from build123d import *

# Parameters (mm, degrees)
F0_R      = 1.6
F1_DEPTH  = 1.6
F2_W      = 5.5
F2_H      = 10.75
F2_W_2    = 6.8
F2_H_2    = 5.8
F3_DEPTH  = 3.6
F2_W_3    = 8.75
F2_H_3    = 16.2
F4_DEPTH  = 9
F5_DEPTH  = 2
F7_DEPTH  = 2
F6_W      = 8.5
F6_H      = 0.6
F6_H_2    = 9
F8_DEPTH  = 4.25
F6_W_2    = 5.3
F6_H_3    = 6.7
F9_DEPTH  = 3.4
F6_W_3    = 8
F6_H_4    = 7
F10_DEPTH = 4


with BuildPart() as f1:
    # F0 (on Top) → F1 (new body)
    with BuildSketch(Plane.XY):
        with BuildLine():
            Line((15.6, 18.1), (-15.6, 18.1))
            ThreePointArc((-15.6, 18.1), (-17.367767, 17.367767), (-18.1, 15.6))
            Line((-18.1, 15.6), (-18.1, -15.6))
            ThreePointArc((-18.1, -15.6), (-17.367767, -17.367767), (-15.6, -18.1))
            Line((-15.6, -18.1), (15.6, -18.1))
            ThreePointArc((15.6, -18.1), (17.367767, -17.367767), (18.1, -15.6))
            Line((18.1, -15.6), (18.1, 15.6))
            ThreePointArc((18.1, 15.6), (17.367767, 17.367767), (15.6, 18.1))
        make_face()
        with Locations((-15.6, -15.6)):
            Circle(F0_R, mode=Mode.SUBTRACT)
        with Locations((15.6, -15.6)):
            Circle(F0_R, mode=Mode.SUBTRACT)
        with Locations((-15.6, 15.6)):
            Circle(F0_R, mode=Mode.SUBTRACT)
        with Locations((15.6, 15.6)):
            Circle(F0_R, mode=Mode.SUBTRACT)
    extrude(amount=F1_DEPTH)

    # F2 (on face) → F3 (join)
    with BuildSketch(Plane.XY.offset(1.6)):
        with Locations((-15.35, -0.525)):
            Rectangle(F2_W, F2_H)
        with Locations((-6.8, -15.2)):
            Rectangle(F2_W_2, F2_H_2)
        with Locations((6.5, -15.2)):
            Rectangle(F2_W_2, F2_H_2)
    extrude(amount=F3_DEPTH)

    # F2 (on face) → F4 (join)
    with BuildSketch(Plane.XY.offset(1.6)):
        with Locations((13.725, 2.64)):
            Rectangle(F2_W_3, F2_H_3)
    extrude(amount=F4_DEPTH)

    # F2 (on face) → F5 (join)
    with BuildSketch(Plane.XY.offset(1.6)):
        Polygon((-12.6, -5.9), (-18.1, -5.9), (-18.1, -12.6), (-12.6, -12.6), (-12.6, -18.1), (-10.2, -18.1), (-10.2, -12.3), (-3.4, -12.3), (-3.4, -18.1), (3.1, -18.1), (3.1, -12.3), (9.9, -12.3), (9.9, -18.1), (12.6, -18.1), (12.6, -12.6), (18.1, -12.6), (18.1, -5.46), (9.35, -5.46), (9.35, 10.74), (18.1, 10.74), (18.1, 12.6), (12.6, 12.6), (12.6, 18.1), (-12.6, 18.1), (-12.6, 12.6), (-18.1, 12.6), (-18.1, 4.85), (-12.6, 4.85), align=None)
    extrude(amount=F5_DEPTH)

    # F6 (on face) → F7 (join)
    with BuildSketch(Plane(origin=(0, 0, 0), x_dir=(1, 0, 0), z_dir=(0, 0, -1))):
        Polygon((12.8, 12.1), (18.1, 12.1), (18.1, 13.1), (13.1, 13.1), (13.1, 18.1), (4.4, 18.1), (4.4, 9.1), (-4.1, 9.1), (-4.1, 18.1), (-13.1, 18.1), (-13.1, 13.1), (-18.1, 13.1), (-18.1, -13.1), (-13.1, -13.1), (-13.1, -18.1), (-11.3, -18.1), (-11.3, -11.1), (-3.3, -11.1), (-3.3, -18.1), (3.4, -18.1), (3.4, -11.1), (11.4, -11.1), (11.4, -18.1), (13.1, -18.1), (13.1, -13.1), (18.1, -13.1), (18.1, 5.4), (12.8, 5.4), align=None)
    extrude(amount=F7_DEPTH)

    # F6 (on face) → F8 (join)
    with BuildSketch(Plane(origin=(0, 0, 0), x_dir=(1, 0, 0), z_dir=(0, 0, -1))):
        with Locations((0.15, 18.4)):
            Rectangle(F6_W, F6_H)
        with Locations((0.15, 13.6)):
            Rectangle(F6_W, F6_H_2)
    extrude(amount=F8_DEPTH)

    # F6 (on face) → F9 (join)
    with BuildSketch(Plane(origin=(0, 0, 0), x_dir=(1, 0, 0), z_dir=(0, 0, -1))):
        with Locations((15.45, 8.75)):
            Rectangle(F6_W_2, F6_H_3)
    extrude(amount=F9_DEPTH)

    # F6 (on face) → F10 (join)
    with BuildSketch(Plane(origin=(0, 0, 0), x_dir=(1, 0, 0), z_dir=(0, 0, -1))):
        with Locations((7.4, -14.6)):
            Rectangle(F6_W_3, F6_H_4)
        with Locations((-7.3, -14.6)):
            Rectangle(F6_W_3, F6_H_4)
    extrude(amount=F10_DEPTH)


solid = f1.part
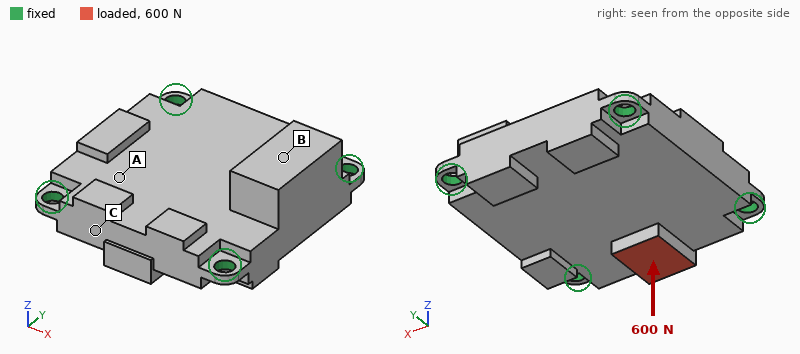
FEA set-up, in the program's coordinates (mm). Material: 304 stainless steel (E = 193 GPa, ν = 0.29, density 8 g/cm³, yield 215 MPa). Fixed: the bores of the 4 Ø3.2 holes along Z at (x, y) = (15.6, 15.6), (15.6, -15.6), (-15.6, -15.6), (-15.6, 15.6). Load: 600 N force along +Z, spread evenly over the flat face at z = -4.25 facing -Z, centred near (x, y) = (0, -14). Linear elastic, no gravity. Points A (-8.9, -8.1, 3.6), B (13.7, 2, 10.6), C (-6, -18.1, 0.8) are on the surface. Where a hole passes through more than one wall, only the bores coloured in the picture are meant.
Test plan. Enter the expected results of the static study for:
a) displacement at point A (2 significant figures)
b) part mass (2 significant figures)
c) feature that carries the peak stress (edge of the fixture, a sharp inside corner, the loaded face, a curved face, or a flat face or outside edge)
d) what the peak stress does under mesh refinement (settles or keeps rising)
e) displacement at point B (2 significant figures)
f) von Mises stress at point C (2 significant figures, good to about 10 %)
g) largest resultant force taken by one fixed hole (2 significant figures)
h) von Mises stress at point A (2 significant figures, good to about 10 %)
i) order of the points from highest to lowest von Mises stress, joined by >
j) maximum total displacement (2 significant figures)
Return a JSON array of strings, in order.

["2.5 µm", "68 g", "edge of the fixture", "keeps rising", "1.7 µm", "21 MPa", "300 N", "14 MPa", "C > A > B", "6.0 µm"]
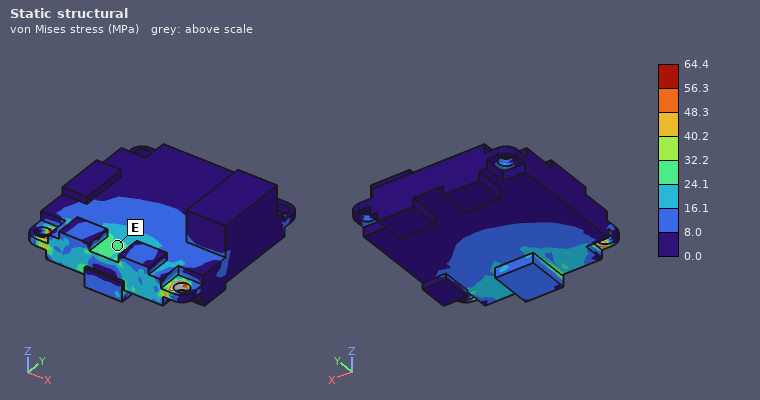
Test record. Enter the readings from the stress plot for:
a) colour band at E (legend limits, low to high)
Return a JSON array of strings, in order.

["24.1 to 32.2 MPa"]
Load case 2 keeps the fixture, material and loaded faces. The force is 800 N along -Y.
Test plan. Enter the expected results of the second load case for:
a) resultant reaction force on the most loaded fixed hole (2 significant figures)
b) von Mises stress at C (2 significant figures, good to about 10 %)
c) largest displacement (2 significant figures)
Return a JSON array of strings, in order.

["240 N", "20 MPa", "5.4 µm"]
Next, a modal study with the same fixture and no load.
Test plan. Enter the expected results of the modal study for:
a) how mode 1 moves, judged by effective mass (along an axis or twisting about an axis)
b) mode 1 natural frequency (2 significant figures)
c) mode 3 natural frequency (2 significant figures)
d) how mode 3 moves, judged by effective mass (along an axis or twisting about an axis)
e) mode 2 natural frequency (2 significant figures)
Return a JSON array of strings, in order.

["along Z", "12 kHz", "19 kHz", "twisting about X", "17 kHz"]
